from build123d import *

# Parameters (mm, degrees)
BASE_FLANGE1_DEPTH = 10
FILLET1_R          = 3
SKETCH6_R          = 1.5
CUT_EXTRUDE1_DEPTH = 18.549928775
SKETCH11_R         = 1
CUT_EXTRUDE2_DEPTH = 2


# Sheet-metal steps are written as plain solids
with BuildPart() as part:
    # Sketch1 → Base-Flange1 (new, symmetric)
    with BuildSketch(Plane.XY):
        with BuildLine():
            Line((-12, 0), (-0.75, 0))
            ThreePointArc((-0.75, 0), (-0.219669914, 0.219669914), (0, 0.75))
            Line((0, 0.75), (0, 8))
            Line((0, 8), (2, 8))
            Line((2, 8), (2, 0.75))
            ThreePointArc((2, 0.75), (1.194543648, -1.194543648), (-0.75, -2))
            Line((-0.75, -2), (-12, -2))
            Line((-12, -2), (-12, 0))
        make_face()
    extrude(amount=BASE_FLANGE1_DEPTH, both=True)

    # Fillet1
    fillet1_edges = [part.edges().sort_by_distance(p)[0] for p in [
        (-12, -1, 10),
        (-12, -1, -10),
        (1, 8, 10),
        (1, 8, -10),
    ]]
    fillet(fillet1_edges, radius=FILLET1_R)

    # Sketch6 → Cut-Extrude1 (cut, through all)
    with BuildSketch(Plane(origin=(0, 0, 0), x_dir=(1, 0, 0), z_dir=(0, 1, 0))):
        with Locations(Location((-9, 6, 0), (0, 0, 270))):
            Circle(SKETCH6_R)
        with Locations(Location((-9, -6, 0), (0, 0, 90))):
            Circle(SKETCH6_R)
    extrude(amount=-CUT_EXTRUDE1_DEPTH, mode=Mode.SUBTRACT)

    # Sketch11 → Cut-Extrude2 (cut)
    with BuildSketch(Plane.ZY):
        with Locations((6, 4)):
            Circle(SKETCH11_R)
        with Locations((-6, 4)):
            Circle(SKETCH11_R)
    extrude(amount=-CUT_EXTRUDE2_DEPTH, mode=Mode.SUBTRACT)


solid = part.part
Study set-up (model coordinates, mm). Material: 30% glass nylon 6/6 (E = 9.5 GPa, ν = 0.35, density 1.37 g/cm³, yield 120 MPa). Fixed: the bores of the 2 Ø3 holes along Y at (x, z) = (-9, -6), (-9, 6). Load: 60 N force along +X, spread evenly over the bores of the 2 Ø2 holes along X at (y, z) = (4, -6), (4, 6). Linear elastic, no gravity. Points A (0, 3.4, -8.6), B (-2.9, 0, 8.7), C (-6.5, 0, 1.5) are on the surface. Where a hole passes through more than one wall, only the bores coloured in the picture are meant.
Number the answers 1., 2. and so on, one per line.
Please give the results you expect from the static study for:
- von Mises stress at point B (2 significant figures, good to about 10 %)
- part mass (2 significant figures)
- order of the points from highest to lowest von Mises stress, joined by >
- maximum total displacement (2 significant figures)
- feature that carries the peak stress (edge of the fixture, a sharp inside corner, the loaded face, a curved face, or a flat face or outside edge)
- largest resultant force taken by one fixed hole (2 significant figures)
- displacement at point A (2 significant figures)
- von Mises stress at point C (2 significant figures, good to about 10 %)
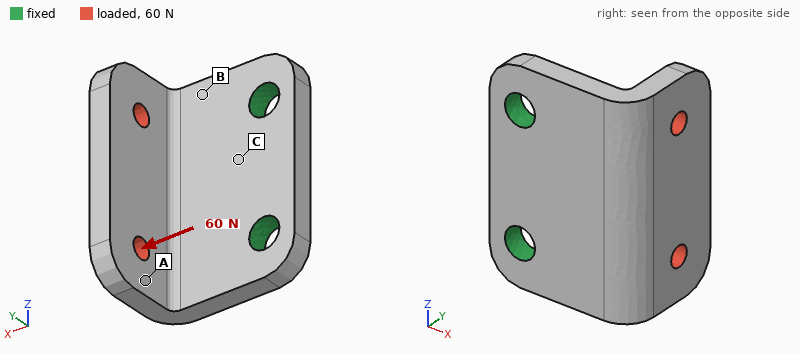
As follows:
1. 23 MPa
2. 1.1 g
3. B > C > A
4. 0.25 mm
5. a flat face or outside edge
6. 31 N
7. 0.13 mm
8. 16 MPa
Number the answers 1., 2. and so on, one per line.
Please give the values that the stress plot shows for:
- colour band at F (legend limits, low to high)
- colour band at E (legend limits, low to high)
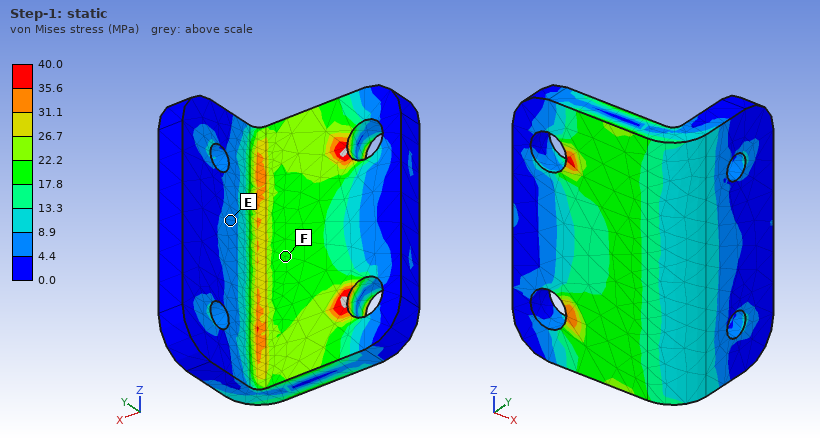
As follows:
1. 17.8 to 22.2 MPa
2. 4.4 to 8.9 MPa
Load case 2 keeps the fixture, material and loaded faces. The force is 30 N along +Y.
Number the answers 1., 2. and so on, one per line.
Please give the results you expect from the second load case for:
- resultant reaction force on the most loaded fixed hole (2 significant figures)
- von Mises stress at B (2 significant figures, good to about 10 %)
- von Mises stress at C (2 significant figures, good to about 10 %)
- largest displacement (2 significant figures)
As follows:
1. 15 N
2. 8.8 MPa
3. 10 MPa
4. 0.12 mm
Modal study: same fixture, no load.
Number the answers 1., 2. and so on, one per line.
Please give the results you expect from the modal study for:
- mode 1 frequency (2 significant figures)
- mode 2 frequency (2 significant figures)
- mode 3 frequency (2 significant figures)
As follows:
1. 3600 Hz
2. 6100 Hz
3. 10 kHz
